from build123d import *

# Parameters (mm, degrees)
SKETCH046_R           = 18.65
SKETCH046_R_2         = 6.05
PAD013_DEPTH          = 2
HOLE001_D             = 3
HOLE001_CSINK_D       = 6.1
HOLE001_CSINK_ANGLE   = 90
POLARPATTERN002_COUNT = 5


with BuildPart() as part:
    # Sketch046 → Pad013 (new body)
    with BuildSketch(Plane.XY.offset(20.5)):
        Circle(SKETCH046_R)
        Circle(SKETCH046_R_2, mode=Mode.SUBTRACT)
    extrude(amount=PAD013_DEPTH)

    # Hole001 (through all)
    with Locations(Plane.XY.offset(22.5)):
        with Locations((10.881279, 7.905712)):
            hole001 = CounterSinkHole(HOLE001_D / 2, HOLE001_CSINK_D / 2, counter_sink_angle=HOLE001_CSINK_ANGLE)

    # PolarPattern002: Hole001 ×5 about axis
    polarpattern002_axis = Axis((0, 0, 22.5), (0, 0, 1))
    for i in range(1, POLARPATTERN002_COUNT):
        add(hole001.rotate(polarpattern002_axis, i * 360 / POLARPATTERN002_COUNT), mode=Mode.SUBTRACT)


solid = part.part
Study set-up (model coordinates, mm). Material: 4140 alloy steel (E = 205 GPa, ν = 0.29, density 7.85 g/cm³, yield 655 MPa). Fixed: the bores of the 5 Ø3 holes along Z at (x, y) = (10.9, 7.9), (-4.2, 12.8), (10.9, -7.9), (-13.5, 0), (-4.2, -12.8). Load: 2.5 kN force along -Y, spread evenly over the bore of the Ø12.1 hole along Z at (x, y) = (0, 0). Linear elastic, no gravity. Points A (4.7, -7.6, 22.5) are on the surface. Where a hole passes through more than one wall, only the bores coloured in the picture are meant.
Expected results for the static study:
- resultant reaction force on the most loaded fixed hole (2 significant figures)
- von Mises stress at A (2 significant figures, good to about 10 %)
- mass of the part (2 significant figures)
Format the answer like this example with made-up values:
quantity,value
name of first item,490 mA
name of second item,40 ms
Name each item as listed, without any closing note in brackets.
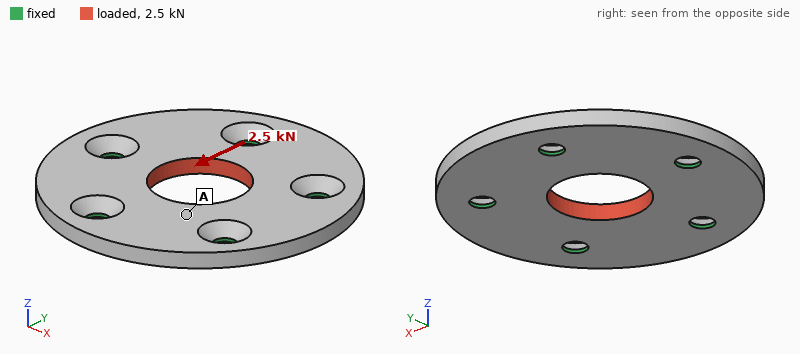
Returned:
quantity,value
resultant reaction force on the most loaded fixed hole,580 N
von Mises stress at A,21 MPa
mass of the part,14 g
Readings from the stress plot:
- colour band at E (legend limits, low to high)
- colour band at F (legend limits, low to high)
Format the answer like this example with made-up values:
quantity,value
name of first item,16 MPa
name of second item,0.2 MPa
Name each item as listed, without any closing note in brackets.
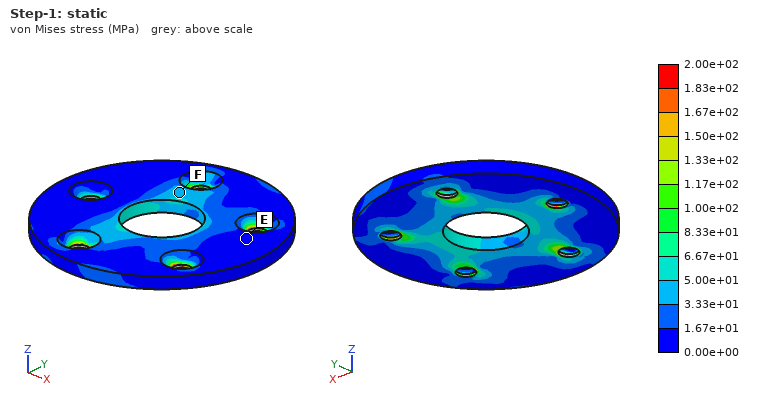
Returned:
quantity,value
colour band at E,0.00e+00 to 1.67e+01 MPa
colour band at F,3.33e+01 to 5.00e+01 MPa
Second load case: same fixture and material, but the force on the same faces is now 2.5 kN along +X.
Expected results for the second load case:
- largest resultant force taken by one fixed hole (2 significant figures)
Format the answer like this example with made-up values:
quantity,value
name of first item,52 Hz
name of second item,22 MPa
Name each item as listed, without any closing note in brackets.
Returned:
quantity,value
largest resultant force taken by one fixed hole,600 N
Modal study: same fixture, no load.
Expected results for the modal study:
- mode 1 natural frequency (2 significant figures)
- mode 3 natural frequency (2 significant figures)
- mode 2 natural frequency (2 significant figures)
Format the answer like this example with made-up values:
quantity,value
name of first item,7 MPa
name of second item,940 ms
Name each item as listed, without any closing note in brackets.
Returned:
quantity,value
mode 1 natural frequency,19 kHz
mode 3 natural frequency,20 kHz
mode 2 natural frequency,19 kHz
